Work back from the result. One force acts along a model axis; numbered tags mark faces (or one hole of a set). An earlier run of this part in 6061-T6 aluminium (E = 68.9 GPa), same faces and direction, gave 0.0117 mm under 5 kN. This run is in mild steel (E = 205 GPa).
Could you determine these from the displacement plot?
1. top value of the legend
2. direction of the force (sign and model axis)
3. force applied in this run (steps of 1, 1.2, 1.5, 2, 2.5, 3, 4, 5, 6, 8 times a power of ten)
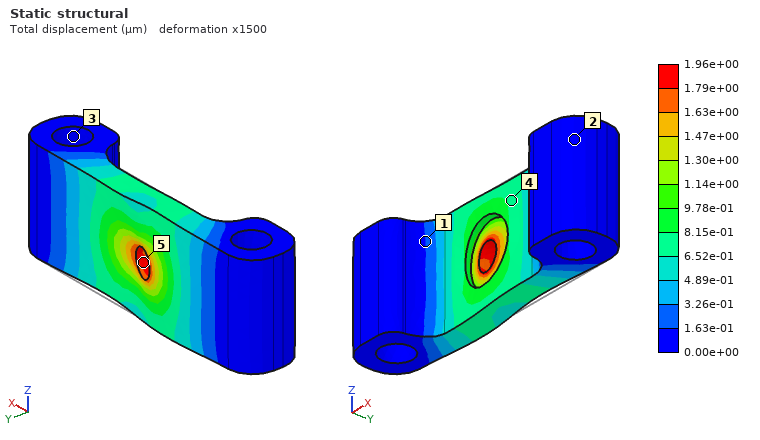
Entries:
1.96e+00 µm
-X
2.5 kN
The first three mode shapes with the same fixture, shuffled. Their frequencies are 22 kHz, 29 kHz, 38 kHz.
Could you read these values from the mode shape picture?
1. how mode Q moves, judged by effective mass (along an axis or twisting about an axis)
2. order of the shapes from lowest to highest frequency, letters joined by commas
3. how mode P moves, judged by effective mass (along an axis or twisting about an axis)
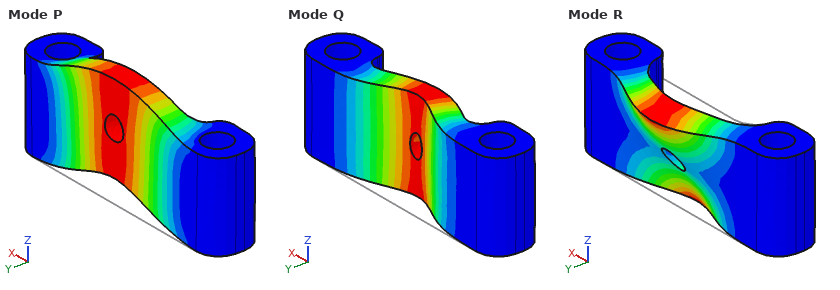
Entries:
along Y
Q, R, P
along Z
